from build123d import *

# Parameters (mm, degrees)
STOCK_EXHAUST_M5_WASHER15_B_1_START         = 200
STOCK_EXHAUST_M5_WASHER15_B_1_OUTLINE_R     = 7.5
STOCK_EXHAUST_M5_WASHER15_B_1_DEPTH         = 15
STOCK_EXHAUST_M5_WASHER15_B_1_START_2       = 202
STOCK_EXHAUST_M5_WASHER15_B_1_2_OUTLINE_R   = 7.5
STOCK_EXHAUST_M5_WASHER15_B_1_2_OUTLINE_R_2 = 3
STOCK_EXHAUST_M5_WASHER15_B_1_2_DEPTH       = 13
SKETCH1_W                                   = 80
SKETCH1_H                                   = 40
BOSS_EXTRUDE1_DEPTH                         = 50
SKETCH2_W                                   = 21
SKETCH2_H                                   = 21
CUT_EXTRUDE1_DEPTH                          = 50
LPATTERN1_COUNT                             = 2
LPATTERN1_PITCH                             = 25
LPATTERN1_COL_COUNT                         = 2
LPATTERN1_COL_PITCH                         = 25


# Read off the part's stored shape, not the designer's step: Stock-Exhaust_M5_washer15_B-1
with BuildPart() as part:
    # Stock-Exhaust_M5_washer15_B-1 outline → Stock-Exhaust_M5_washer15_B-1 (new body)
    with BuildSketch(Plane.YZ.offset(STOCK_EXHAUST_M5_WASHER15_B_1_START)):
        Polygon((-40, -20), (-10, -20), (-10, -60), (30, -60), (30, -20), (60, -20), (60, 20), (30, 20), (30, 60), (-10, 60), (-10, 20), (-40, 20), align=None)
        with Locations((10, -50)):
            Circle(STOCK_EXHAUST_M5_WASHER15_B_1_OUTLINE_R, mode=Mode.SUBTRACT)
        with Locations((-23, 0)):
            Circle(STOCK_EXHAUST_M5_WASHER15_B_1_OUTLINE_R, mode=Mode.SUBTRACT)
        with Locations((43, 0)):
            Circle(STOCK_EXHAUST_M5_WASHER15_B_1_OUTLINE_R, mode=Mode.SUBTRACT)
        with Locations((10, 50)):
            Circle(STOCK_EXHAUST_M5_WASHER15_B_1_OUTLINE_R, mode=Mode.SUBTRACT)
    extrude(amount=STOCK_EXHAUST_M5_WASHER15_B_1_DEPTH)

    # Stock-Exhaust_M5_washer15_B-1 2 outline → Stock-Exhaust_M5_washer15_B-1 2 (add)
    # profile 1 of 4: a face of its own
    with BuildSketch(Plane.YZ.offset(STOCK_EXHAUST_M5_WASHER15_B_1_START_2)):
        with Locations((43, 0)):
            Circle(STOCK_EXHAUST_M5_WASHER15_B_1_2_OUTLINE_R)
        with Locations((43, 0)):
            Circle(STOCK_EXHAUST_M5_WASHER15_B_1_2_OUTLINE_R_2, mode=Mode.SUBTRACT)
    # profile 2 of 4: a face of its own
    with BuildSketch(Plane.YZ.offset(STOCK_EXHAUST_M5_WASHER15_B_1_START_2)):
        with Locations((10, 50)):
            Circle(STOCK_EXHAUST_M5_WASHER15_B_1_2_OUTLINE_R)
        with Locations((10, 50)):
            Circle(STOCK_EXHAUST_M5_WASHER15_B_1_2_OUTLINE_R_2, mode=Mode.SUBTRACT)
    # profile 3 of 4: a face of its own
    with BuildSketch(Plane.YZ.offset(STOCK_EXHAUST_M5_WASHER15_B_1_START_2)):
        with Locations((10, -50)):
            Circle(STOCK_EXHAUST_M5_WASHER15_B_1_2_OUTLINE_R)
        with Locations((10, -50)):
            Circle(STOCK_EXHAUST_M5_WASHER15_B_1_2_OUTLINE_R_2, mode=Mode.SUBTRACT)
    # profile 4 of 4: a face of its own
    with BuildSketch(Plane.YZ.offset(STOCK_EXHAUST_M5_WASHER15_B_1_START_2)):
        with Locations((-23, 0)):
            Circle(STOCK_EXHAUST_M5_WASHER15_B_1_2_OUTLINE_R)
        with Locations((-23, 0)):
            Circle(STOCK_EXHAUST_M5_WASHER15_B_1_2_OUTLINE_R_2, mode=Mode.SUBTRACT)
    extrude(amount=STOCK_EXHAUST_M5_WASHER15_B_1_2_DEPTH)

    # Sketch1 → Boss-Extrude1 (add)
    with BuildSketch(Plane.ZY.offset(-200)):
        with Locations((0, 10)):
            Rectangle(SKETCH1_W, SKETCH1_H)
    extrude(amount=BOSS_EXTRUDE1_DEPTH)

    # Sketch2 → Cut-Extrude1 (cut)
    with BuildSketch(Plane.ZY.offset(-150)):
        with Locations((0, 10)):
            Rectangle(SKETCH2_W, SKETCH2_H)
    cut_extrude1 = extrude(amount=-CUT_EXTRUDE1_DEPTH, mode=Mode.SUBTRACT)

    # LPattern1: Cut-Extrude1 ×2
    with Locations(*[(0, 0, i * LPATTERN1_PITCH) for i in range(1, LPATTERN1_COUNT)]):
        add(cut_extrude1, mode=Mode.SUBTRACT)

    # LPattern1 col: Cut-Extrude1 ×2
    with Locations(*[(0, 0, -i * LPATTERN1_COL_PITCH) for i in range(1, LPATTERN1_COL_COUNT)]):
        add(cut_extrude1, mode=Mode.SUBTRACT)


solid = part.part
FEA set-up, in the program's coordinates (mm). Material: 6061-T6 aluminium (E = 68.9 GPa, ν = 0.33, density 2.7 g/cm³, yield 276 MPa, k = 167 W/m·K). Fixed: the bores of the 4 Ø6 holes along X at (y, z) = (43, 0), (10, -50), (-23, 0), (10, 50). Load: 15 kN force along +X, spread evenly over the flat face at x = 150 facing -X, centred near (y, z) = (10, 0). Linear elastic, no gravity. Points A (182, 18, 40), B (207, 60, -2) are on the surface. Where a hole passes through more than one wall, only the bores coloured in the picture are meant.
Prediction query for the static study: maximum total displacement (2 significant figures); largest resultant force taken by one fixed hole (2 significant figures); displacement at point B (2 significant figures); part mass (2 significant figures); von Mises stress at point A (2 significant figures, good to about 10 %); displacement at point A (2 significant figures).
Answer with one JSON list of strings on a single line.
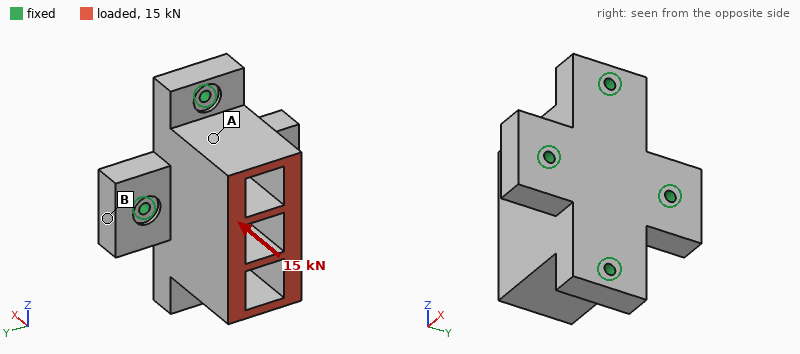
["17 µm", "4.0 kN", "2.8 µm", "540 g", "9.8 MPa", "13 µm"]
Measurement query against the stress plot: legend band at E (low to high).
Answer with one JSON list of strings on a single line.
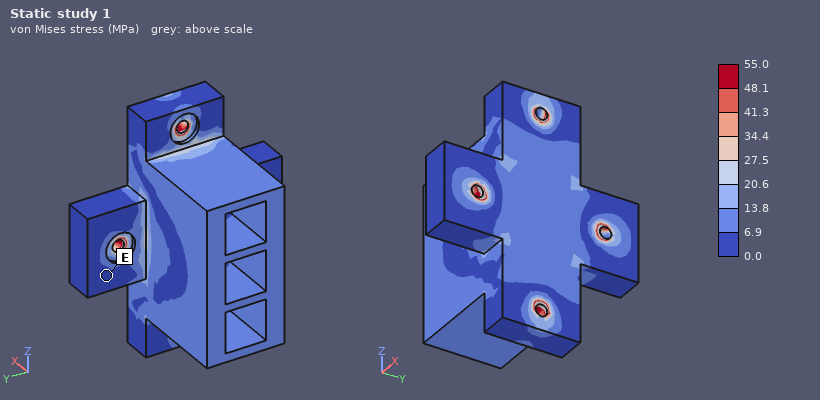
["0.0 to 6.9 MPa"]
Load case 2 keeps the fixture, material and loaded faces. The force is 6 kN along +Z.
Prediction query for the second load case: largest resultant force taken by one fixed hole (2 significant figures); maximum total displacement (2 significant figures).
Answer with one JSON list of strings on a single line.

["4.3 kN", "35 µm"]
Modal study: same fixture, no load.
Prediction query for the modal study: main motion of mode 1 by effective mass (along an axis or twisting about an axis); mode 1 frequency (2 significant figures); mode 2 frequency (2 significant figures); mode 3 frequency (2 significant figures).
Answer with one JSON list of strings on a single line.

["along Y", "4900 Hz", "6800 Hz", "6900 Hz"]
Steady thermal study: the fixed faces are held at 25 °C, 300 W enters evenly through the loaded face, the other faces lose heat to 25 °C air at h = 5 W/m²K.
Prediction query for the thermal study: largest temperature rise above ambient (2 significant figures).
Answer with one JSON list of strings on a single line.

["66 K"]
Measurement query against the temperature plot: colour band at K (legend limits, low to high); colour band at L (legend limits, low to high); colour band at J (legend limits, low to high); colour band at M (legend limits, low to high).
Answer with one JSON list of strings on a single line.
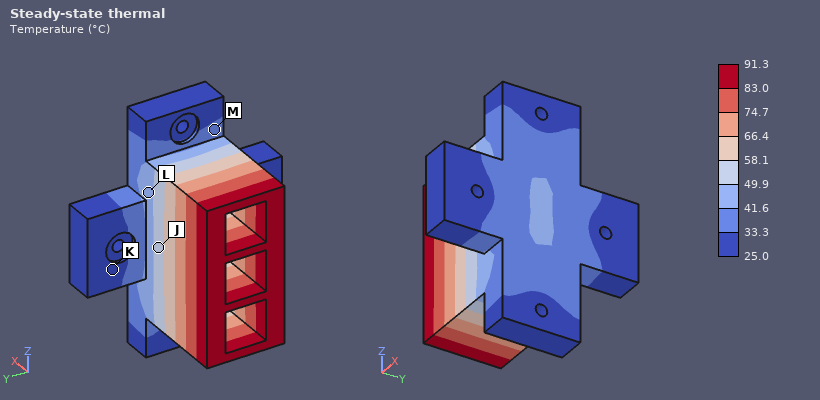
["25.0 to 33.3 °C", "41.6 to 49.9 °C", "49.9 to 58.1 °C", "33.3 to 41.6 °C"]
